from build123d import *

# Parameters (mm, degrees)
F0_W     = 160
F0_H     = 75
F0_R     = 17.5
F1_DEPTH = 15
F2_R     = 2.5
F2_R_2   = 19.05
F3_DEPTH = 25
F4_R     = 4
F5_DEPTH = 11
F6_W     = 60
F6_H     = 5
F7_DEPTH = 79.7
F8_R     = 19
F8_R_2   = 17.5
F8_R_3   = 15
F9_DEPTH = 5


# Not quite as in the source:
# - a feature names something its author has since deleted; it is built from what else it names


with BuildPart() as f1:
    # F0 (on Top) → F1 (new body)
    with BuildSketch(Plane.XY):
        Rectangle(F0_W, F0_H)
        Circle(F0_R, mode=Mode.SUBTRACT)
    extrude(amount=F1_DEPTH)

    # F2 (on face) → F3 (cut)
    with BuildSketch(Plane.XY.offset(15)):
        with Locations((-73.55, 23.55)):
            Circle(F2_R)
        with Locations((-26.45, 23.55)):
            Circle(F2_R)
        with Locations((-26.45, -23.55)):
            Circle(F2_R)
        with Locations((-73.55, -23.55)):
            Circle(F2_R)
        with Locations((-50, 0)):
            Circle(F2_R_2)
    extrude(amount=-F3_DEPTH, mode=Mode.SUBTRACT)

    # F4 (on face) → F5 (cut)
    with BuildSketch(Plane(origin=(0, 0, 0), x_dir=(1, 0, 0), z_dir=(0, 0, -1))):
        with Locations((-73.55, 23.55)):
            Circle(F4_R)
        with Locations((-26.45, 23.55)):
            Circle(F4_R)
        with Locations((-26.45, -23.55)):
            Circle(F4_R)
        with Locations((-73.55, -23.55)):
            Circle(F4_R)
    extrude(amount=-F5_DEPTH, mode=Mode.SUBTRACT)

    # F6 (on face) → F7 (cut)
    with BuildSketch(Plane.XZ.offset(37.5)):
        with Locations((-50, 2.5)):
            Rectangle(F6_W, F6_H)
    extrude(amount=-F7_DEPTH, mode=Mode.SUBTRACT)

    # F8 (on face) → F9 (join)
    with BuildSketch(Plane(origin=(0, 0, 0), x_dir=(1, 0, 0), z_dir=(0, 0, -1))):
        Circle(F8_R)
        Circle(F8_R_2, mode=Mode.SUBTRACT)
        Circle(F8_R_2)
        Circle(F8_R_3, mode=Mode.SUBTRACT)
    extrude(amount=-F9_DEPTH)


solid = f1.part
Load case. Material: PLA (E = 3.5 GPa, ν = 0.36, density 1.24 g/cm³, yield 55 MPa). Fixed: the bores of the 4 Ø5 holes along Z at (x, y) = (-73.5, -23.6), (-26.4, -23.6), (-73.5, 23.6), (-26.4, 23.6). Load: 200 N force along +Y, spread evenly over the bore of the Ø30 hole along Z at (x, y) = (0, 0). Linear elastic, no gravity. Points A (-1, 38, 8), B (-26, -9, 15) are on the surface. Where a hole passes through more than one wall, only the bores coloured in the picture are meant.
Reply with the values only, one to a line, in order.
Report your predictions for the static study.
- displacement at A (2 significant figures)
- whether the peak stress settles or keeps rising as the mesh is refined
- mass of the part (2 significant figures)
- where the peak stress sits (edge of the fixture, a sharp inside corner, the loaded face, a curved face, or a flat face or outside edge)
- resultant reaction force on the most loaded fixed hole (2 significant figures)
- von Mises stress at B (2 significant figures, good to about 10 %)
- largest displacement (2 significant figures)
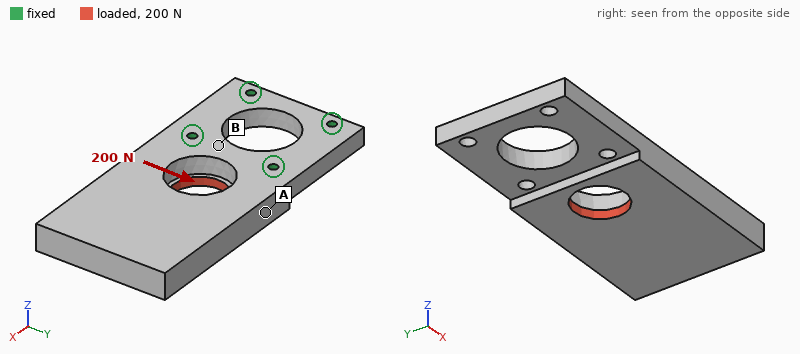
20 µm
keeps rising
160 g
edge of the fixture
130 N
0.69 MPa
36 µm
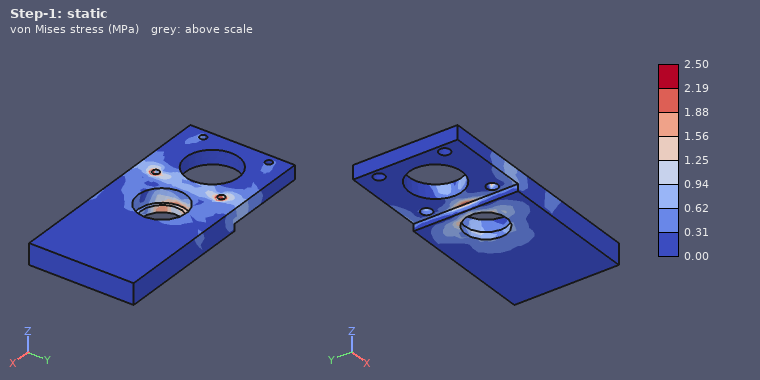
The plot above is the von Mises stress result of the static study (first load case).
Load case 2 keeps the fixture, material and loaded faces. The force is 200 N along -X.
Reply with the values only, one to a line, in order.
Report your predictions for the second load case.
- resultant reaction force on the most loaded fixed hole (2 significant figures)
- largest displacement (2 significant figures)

55 N
0.25 mm
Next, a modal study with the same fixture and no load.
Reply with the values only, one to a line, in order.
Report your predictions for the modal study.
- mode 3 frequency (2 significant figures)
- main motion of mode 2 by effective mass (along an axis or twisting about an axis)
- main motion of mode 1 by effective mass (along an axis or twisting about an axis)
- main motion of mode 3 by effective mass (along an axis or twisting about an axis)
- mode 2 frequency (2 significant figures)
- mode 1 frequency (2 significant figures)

880 Hz
along Y
along Z
along Y
700 Hz
180 Hz
